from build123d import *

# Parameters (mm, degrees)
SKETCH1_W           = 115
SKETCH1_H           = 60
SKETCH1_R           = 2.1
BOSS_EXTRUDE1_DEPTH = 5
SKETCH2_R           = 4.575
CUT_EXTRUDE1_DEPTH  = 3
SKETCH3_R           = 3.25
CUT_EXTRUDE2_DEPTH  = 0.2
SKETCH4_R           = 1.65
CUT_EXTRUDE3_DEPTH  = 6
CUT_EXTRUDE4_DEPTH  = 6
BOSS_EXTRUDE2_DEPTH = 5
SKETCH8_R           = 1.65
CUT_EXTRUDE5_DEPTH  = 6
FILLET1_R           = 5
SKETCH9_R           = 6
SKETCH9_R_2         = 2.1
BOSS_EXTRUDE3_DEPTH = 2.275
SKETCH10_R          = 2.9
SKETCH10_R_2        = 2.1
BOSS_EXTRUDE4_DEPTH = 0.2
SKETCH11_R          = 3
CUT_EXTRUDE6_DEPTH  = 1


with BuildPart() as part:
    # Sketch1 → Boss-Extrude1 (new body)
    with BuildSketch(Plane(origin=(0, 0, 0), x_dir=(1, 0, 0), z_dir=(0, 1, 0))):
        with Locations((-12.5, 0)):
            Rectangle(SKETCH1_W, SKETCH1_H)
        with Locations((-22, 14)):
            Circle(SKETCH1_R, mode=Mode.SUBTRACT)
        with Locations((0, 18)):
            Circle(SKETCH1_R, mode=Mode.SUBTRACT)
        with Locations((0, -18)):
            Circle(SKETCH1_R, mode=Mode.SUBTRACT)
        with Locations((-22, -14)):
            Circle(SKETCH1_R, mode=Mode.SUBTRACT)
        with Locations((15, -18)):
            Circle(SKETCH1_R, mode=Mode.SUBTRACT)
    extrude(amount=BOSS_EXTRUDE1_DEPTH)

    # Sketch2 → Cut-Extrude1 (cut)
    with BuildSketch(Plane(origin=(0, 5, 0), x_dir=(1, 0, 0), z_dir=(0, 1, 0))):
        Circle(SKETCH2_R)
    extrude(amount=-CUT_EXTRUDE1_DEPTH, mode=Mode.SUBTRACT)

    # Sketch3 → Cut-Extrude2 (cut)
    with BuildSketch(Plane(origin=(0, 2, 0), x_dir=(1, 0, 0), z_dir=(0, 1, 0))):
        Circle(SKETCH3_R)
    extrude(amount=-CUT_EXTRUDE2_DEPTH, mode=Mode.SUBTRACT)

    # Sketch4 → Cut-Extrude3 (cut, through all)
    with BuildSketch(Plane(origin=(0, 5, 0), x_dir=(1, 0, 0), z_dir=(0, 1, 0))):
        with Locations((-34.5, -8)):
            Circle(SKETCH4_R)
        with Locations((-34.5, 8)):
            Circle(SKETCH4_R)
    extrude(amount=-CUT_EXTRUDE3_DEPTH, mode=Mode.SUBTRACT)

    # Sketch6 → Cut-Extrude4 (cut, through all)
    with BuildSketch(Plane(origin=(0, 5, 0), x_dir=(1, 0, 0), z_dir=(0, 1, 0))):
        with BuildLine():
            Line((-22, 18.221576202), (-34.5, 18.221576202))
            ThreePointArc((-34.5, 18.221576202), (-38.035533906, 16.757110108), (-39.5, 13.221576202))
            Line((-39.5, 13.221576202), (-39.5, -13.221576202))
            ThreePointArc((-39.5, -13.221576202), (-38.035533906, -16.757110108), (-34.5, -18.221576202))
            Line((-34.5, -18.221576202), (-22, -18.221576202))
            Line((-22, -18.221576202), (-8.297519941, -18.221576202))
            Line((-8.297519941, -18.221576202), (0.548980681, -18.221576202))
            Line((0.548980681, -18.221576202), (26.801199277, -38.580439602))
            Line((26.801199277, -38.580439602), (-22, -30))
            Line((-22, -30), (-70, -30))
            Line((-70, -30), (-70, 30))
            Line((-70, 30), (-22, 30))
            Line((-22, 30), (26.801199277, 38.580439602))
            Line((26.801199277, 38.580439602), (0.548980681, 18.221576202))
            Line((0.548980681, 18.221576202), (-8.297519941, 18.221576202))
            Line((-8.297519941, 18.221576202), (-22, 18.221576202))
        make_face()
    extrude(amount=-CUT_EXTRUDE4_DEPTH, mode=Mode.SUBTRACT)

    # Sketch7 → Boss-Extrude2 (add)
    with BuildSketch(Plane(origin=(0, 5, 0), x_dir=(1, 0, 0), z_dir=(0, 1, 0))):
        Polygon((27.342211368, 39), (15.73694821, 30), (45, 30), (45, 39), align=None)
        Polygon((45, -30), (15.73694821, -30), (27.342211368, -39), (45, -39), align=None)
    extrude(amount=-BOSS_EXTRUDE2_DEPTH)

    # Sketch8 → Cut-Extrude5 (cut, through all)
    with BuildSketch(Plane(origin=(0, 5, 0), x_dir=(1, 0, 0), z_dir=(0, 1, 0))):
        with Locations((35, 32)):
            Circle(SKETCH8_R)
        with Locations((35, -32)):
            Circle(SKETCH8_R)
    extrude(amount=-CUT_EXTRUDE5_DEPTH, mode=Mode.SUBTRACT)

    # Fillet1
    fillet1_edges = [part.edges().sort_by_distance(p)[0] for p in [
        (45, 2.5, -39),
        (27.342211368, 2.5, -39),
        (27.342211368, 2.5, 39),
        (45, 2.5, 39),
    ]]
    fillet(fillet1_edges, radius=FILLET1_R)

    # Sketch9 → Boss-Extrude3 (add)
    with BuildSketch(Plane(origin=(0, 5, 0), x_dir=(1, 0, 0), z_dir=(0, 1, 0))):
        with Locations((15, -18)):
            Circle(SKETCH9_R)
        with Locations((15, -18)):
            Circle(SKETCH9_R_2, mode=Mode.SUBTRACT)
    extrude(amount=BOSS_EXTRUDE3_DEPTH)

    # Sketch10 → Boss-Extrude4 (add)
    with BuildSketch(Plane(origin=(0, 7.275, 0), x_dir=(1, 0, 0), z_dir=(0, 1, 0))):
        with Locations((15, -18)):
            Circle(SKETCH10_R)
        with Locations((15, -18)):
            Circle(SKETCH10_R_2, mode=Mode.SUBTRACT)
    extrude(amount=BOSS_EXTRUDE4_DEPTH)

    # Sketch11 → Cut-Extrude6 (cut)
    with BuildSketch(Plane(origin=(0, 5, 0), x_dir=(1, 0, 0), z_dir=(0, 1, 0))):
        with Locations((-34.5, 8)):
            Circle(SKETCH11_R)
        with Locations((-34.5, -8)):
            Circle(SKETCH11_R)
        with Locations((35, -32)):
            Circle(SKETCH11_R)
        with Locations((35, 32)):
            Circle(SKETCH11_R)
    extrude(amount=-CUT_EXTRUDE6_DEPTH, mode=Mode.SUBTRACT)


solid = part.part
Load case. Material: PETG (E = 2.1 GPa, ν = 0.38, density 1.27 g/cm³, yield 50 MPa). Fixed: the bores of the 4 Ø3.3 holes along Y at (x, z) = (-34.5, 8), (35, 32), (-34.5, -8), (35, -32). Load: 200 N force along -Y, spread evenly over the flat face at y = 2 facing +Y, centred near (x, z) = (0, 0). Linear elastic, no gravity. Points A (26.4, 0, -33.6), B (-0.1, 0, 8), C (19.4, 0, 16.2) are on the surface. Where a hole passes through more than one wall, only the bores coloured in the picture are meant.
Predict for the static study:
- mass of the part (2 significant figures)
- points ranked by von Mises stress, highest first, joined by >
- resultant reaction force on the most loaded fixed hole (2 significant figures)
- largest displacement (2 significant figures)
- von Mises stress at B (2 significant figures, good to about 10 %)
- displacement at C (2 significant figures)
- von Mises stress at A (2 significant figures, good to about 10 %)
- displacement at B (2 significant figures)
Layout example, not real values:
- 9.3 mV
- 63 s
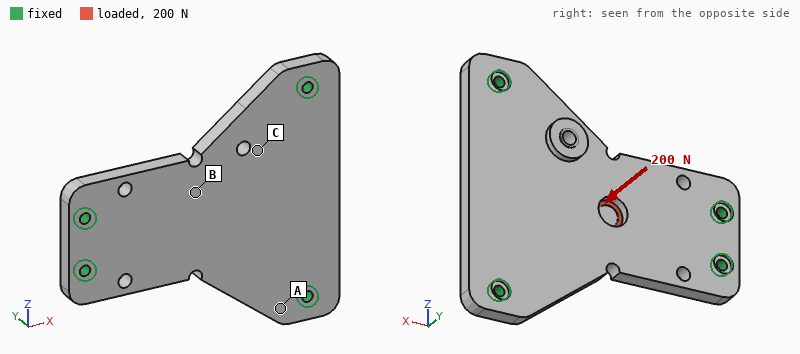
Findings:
- 27 g
- B > A > C
- 54 N
- 0.72 mm
- 12 MPa
- 0.35 mm
- 5.0 MPa
- 0.65 mm
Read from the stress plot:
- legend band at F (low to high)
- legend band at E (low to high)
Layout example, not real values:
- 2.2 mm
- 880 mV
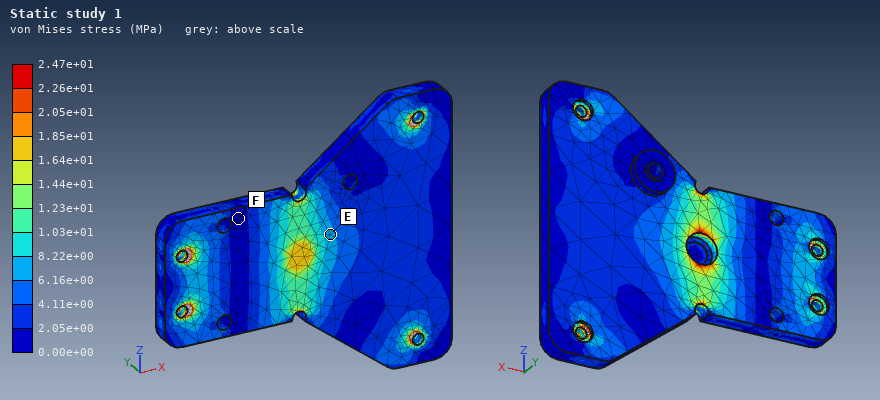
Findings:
- 0.00e+00 to 2.05e+00 MPa
- 6.16e+00 to 8.22e+00 MPa
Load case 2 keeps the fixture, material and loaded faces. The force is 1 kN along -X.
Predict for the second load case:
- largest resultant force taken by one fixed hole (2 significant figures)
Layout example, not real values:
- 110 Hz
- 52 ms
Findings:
- 300 N
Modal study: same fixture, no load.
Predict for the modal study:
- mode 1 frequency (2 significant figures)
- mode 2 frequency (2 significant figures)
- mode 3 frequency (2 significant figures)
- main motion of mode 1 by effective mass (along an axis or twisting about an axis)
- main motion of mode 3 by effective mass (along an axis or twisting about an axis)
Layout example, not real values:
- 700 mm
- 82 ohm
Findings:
- 970 Hz
- 1600 Hz
- 1800 Hz
- along Y
- twisting about X
